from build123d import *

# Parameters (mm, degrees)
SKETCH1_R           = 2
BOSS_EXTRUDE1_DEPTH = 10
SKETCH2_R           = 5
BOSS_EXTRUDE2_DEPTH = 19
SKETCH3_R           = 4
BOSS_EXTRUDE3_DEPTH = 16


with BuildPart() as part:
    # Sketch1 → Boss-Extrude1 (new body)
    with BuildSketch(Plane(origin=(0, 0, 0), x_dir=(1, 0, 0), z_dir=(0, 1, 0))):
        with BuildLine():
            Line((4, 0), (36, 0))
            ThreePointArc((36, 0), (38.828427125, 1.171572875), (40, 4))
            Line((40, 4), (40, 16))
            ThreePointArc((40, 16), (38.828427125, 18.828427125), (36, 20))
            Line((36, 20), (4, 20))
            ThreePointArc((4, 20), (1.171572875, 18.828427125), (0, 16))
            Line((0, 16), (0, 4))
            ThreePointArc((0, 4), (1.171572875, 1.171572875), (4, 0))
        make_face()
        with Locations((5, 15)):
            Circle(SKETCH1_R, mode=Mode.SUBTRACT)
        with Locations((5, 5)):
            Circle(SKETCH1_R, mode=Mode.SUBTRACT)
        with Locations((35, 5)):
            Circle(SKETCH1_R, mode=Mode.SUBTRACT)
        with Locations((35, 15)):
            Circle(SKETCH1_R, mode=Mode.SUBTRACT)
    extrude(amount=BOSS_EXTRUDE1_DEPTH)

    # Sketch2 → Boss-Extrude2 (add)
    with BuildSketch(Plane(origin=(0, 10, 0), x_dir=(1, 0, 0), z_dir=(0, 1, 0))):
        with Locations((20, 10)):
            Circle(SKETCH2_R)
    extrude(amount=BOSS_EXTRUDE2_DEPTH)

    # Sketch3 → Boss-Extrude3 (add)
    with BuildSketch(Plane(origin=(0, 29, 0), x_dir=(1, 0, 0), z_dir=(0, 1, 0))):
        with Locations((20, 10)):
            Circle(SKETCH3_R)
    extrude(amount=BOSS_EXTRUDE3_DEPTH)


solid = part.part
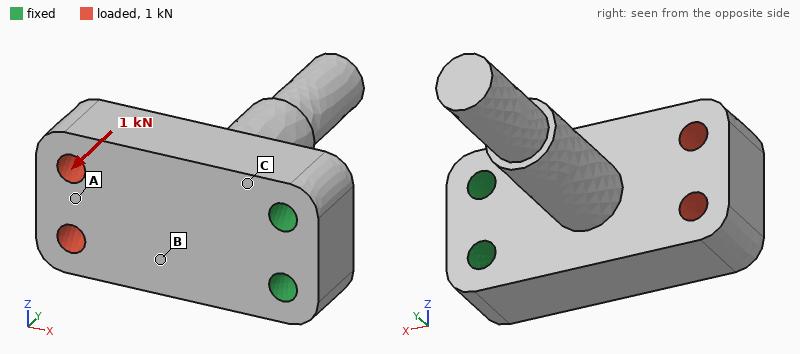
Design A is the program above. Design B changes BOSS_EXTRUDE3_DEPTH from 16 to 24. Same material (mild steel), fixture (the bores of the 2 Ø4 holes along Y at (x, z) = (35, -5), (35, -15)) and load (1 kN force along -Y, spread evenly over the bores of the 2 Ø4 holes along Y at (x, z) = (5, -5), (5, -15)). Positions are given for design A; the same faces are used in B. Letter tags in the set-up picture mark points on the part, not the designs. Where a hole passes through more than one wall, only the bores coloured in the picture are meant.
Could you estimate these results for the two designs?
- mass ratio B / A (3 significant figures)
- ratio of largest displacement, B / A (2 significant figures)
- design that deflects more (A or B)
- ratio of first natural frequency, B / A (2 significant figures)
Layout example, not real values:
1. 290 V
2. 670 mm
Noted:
1. 1.04
2. 1.2
3. B
4. 0.75
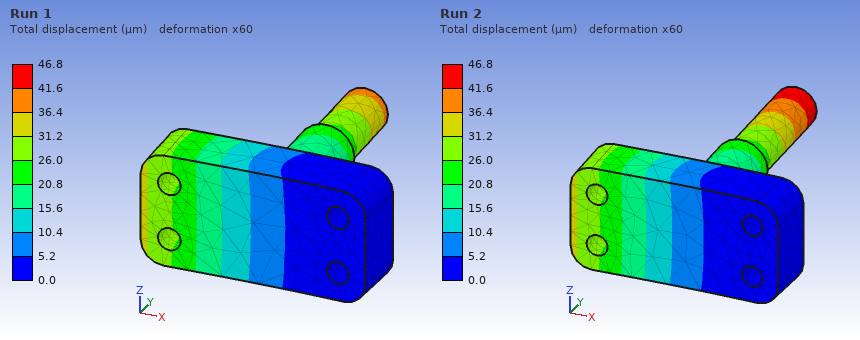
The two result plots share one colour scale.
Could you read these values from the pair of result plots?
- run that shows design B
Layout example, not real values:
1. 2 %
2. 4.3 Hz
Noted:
1. Run 2
